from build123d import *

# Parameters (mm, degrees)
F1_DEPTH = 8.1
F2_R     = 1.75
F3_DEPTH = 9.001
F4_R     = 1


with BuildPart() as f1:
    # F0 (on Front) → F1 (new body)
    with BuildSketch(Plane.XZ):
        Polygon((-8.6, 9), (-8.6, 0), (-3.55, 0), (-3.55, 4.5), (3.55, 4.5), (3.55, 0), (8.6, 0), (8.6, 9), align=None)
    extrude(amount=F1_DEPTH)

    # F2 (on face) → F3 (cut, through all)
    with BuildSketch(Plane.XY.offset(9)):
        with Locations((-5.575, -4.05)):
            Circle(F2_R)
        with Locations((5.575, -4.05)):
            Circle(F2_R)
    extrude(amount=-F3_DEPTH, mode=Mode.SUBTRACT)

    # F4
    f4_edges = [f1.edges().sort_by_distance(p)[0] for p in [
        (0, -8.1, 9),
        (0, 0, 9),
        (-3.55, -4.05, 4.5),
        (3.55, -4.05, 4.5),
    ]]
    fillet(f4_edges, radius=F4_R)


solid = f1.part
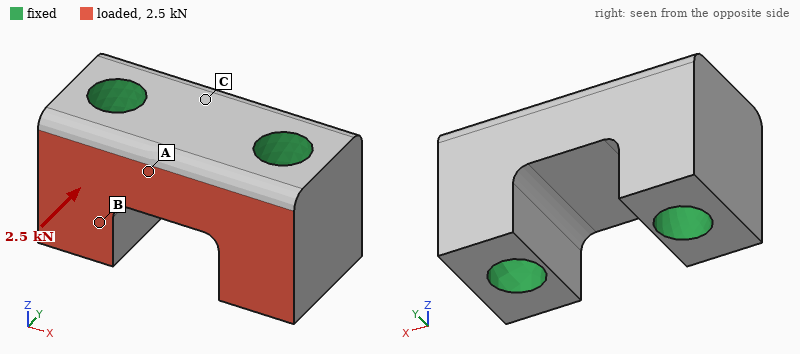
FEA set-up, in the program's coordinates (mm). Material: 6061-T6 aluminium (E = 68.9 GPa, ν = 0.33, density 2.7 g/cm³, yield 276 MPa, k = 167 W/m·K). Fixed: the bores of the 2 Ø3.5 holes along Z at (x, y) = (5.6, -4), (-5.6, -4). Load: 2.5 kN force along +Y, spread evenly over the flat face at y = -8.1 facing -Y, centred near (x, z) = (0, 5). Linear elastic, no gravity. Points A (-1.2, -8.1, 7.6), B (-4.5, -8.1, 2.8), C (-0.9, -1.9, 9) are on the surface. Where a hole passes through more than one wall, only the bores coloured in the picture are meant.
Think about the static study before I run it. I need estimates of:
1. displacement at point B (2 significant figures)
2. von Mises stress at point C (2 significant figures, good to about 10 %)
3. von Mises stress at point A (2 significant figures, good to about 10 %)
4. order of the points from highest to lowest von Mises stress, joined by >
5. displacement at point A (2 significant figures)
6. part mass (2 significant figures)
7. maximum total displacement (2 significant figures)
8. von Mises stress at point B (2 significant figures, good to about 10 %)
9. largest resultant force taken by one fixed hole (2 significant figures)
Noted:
0.85 µm
6.1 MPa
13 MPa
B > A > C
1.6 µm
2.2 g
2.3 µm
25 MPa
1.3 kN
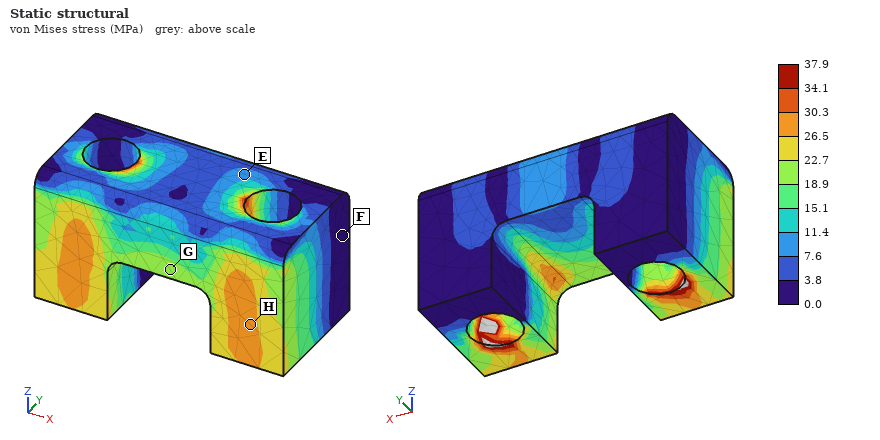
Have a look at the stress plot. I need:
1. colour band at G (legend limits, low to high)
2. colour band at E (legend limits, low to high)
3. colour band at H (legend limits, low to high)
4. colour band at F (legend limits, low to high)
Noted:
18.9 to 22.7 MPa
7.6 to 11.4 MPa
26.5 to 30.3 MPa
0.0 to 3.8 MPa
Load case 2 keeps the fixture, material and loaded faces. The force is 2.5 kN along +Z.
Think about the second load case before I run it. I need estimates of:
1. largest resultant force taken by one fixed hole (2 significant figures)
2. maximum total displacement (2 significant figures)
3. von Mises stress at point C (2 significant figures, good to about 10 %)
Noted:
1.3 kN
7.5 µm
9.6 MPa
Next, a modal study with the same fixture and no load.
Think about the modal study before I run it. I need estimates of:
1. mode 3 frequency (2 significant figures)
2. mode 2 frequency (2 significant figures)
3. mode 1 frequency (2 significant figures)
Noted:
150 kHz
150 kHz
150 kHz
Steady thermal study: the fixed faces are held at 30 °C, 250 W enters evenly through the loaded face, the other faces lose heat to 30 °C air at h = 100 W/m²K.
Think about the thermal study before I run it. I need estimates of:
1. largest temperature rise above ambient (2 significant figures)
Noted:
51 K
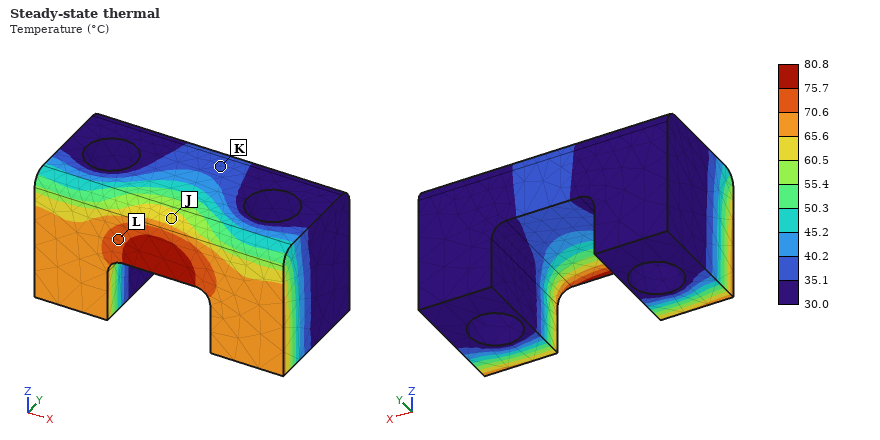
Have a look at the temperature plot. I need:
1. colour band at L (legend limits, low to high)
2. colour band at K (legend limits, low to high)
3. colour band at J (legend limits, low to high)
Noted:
70.6 to 75.7 °C
35.1 to 40.2 °C
60.5 to 65.6 °C
